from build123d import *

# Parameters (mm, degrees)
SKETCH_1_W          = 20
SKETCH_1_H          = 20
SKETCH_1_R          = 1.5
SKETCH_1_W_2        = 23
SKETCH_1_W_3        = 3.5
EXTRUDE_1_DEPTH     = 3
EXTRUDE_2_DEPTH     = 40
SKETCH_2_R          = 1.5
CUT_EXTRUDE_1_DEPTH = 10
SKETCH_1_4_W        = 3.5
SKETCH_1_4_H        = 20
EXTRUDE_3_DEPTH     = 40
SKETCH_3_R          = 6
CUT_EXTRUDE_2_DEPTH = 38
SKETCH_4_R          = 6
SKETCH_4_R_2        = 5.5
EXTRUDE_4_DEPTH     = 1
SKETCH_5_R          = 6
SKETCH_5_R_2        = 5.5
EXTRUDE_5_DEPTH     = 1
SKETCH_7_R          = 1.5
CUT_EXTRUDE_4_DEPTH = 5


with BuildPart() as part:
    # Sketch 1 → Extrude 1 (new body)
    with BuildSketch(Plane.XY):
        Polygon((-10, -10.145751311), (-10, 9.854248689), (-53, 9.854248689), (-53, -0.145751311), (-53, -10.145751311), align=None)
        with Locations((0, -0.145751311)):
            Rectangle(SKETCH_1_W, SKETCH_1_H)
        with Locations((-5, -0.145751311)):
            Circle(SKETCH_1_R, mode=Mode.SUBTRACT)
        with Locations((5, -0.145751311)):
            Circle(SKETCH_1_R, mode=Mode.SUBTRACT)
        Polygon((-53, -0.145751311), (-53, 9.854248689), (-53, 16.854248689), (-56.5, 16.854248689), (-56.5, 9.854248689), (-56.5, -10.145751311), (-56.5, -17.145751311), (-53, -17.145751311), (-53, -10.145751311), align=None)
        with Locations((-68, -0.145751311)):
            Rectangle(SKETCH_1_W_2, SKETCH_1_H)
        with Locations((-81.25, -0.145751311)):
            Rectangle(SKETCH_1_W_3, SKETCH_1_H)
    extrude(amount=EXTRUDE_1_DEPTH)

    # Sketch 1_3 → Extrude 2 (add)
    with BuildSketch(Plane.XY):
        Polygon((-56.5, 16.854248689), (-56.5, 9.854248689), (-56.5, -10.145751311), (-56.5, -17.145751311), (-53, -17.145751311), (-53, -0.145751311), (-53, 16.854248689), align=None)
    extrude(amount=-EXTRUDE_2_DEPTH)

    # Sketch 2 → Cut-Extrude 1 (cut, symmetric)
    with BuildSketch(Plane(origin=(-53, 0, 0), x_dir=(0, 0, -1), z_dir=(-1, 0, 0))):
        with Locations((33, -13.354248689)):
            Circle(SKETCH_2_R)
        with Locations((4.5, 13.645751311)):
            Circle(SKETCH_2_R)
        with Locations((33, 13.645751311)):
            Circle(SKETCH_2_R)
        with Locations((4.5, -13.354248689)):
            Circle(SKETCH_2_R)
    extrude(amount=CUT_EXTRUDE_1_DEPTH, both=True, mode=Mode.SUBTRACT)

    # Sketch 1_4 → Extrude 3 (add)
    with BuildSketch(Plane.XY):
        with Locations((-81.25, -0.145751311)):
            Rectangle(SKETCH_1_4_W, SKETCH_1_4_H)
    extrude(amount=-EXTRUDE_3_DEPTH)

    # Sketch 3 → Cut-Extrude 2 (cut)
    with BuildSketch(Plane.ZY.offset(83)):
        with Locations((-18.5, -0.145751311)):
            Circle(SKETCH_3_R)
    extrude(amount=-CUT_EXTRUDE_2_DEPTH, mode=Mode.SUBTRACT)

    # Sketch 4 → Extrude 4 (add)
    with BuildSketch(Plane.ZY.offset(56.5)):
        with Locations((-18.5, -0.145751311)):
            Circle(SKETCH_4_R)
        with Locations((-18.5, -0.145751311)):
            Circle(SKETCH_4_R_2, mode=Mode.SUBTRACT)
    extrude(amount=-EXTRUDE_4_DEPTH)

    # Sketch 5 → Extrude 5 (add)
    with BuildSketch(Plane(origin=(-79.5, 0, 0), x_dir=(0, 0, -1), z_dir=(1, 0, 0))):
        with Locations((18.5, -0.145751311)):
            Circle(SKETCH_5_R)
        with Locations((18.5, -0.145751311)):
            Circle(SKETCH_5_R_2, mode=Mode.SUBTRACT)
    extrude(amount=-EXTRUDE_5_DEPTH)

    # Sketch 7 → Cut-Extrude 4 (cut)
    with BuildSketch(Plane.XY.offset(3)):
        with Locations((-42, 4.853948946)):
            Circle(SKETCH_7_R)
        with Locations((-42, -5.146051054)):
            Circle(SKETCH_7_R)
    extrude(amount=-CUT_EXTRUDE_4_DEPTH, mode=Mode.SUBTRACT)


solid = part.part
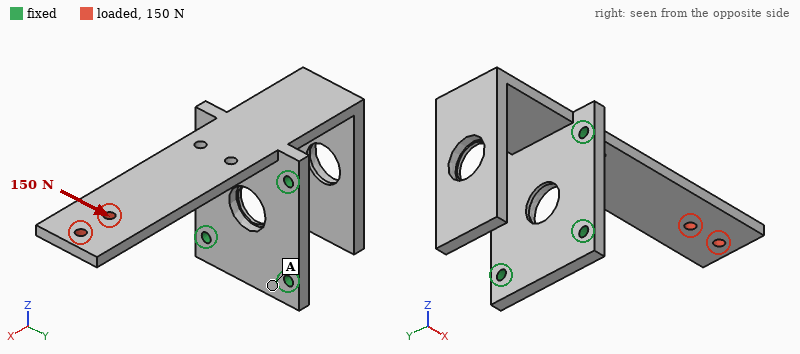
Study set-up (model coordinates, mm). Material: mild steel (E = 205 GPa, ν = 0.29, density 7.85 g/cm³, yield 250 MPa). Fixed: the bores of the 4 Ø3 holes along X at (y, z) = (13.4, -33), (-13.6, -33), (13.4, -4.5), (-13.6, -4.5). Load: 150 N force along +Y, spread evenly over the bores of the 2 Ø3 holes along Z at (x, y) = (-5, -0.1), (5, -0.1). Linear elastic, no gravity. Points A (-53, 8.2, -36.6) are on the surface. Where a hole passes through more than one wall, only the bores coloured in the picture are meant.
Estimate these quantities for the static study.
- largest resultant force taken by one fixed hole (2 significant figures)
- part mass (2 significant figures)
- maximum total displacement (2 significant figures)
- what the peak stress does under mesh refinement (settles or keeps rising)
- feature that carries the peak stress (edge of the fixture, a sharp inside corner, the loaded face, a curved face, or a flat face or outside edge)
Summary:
370 N
97 g
52 µm
keeps rising
edge of the fixture
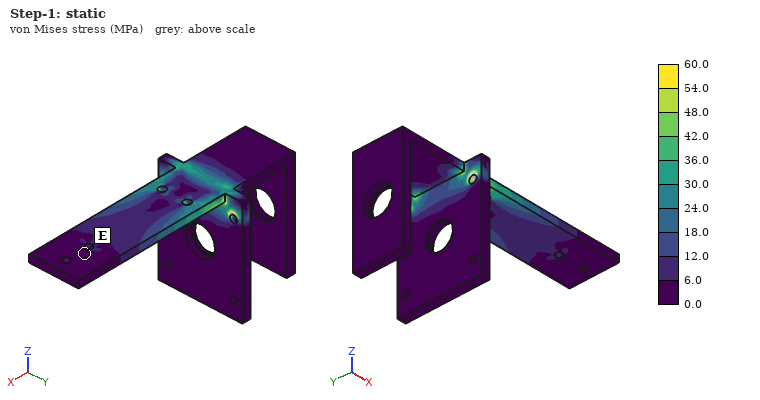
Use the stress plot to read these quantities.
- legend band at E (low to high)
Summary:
0.0 to 6.0 MPa
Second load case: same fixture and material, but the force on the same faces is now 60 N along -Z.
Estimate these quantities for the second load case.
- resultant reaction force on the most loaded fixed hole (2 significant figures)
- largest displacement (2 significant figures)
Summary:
27 N
0.52 mm
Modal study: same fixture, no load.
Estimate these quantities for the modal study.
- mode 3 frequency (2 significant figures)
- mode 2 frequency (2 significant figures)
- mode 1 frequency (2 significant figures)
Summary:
1100 Hz
690 Hz
540 Hz
